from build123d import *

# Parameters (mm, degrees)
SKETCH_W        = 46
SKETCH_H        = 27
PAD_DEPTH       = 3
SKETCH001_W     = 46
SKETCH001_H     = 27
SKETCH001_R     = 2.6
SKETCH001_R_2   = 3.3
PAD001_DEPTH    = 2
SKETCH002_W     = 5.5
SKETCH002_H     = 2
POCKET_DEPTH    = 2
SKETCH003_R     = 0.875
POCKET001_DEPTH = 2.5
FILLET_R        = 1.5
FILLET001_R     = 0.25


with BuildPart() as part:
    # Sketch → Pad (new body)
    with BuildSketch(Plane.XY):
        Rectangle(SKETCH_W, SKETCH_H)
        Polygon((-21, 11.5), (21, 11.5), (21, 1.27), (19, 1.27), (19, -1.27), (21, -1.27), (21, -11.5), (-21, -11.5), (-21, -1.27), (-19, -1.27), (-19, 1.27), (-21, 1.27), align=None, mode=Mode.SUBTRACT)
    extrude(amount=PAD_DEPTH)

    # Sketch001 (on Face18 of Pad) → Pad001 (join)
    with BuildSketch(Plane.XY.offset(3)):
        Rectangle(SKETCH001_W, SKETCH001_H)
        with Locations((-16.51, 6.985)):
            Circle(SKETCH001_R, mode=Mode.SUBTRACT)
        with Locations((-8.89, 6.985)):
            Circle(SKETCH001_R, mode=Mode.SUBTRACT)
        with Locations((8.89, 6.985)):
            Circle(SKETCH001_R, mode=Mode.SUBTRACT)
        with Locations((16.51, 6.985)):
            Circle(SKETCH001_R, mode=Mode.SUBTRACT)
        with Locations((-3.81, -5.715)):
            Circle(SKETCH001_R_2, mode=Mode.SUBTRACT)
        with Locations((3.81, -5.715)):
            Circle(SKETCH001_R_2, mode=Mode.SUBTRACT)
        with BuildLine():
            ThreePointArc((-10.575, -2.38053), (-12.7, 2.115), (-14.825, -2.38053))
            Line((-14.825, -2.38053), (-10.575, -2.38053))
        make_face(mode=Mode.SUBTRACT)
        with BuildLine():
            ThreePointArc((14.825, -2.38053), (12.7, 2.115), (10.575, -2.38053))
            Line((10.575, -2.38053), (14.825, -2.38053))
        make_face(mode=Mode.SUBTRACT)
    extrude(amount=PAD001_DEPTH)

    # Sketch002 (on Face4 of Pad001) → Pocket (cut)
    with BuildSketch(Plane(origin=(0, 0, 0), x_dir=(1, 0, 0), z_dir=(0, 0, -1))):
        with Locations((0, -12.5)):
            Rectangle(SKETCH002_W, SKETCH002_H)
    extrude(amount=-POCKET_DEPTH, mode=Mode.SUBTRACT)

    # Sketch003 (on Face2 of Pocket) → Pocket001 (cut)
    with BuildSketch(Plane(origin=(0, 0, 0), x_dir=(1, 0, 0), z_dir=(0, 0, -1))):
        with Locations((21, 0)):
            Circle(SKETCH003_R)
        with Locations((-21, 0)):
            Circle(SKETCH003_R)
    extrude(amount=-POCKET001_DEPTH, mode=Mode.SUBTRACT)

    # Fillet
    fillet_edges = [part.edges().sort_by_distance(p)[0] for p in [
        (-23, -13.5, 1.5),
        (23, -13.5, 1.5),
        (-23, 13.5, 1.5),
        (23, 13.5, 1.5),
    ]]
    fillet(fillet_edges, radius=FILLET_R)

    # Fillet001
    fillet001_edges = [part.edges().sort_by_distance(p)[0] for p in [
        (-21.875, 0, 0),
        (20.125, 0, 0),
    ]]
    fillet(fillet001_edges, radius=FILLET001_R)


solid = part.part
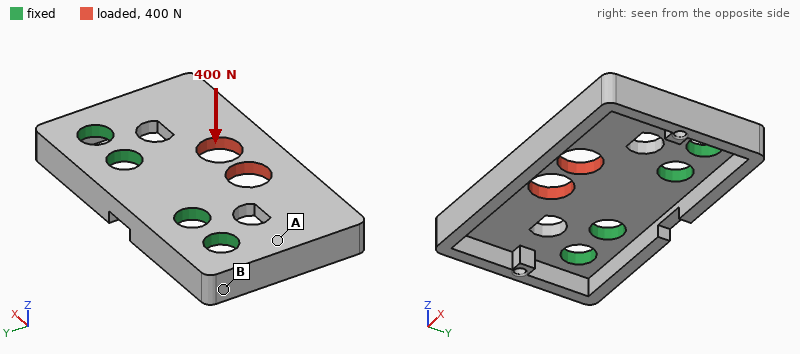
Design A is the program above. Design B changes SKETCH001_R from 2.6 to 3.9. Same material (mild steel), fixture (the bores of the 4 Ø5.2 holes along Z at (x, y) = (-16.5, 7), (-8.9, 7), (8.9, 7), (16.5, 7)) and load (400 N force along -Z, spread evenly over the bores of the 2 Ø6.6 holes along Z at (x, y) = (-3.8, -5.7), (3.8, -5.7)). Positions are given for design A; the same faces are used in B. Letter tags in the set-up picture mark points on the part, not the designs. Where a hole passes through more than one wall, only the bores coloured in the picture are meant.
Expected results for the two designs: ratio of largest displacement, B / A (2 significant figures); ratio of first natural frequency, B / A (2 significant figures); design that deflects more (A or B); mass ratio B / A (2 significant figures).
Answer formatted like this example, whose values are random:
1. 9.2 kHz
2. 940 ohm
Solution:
1. 0.76
2. 1.2
3. A
4. 0.93
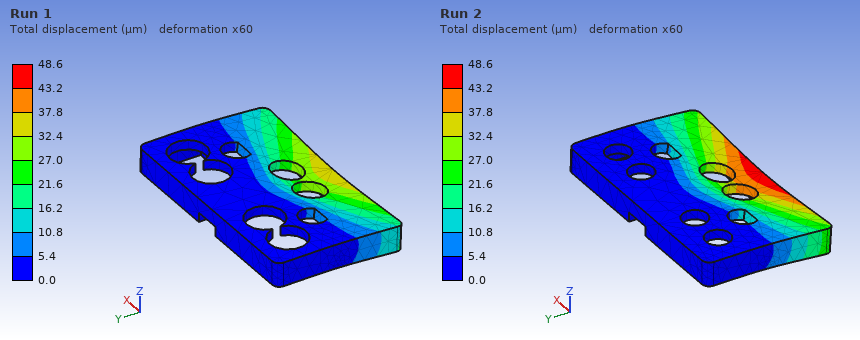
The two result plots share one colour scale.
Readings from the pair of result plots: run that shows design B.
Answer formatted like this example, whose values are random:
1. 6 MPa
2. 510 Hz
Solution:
1. Run 1
